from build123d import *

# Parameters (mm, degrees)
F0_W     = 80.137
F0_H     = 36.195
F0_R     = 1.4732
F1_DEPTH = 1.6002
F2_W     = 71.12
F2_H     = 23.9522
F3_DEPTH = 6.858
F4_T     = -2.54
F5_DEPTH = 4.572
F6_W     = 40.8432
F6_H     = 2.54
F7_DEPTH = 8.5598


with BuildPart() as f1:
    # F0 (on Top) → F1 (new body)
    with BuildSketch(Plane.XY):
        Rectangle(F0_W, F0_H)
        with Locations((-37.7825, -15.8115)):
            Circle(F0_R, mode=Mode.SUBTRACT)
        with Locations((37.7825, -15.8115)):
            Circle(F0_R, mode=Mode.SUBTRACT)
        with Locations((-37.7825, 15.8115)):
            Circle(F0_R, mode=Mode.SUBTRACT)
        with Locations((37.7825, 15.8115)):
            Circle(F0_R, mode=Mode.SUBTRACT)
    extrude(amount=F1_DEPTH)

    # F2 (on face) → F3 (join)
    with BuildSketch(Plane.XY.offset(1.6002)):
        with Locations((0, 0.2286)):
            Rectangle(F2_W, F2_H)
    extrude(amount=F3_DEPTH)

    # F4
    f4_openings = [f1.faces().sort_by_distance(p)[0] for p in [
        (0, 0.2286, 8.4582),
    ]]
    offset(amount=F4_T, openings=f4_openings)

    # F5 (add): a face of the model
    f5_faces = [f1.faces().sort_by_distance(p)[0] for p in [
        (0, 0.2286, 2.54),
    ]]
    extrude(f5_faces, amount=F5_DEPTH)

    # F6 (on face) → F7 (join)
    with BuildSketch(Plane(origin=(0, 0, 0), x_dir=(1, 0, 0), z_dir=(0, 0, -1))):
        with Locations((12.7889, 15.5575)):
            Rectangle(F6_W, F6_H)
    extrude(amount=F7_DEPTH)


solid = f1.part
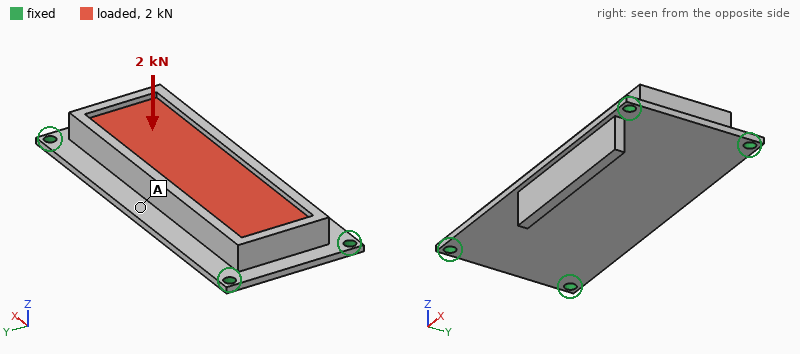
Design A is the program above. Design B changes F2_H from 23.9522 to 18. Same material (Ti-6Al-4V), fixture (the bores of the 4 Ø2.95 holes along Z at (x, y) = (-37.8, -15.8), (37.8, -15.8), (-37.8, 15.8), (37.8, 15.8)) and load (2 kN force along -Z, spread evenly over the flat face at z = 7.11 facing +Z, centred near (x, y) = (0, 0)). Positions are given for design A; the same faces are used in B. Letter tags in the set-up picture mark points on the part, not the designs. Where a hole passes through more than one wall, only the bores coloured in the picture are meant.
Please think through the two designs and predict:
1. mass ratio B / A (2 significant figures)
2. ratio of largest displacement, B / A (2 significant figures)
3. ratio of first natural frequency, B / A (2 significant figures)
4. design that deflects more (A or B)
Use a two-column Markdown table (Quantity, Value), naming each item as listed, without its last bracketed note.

| Quantity | Value |
|---|---|
| mass ratio B / A | 0.85 |
| ratio of largest displacement, B / A | 1.6 |
| ratio of first natural frequency, B / A | 0.86 |
| design that deflects more | B |
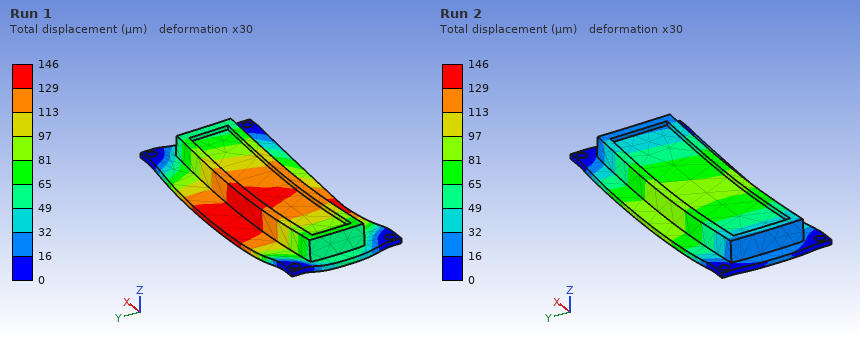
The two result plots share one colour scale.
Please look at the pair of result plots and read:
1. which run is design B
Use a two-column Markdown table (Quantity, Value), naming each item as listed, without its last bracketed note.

| Quantity | Value |
|---|---|
| which run is design B | Run 1 |
